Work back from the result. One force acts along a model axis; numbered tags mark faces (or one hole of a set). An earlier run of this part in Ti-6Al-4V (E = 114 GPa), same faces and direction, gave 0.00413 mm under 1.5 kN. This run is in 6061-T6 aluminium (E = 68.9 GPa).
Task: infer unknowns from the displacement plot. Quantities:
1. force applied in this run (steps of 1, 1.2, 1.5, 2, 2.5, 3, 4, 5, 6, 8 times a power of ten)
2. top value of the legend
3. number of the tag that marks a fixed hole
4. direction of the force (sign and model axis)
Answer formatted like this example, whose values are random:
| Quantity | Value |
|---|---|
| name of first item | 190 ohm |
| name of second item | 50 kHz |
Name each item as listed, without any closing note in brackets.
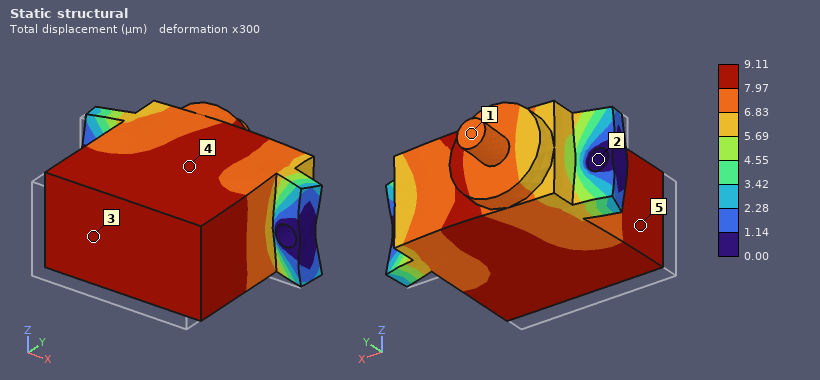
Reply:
| Quantity | Value |
|---|---|
| force applied in this run | 2 kN |
| top value of the legend | 9.11 µm |
| number of the tag that marks a fixed hole | 2 |
| direction of the force | +Y |
